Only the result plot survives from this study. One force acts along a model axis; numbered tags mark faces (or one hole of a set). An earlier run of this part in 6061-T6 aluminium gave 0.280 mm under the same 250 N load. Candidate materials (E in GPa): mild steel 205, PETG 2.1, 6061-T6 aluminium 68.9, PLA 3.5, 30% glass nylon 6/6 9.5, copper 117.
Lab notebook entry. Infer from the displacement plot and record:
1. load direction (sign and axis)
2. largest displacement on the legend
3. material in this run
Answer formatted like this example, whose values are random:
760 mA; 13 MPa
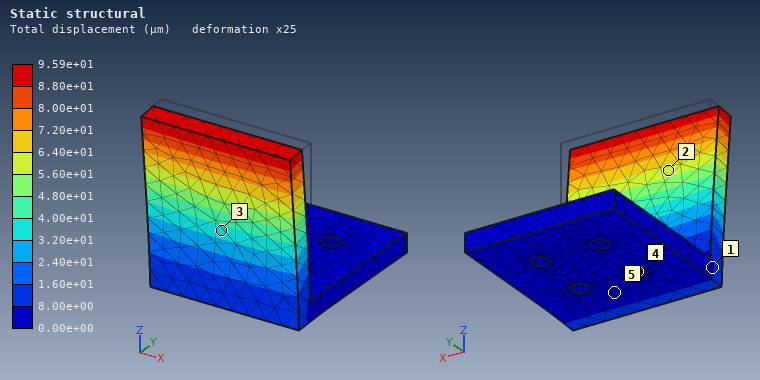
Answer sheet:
-Y; 9.59e+01 µm; mild steel
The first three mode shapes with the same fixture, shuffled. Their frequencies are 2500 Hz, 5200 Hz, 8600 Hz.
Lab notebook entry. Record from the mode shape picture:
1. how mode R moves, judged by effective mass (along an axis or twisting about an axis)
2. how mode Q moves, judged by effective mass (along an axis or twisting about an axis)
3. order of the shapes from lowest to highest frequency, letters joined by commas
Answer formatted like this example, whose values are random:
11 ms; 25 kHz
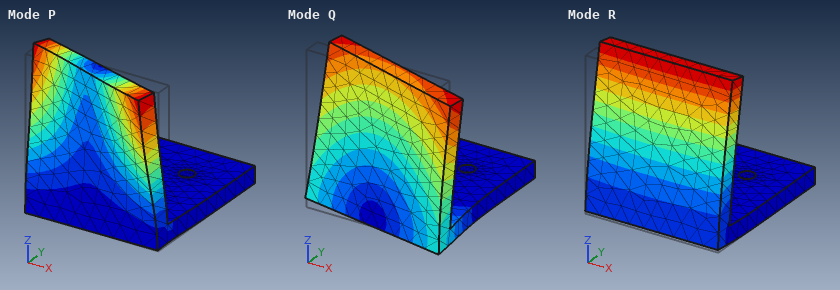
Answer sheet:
along Y; along X; R, Q, P
